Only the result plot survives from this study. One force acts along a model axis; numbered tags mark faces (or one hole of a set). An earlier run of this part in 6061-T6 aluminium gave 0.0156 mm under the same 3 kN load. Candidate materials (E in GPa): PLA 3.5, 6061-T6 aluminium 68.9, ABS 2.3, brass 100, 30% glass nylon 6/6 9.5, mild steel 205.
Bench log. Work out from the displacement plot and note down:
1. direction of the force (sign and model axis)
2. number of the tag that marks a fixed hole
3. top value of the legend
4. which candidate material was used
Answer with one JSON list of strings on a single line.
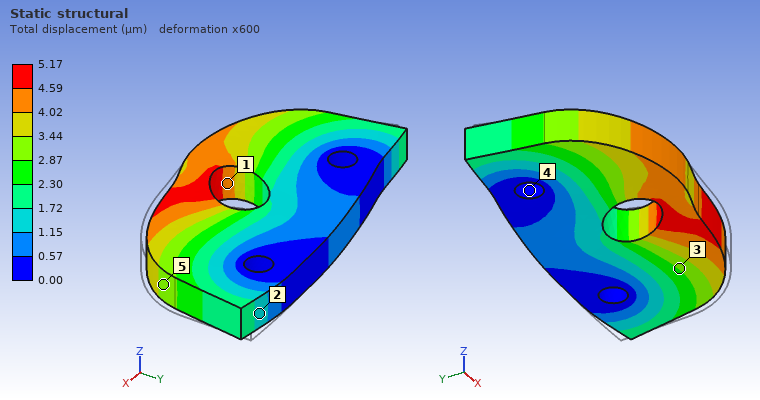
["-X", "4", "5.17 µm", "mild steel"]
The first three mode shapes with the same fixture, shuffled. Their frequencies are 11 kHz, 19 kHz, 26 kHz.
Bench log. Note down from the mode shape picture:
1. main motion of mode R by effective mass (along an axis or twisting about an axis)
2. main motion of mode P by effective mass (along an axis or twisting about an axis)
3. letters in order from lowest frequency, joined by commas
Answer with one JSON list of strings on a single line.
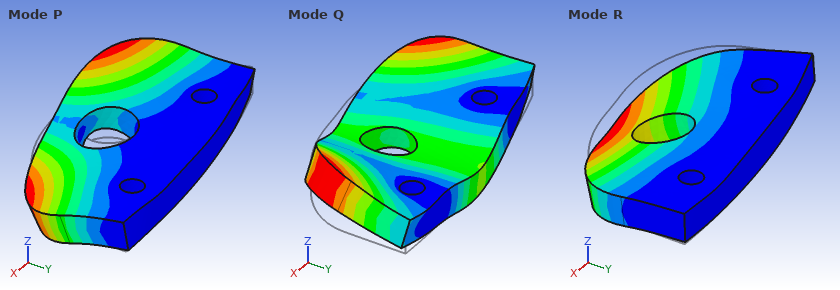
["along Z", "twisting about Y", "R, P, Q"]
